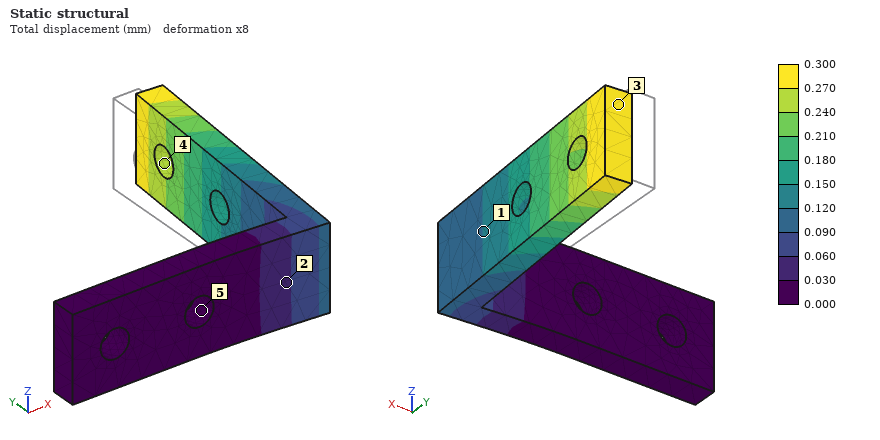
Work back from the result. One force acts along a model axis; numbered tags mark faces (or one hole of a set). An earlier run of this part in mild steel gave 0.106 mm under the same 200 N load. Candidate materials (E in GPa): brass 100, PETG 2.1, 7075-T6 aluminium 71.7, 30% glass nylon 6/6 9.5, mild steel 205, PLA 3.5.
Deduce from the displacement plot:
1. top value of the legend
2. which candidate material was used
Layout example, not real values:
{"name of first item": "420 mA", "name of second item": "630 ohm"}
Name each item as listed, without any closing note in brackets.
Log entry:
{"top value of the legend": "0.300 mm", "which candidate material was used": "7075-T6 aluminium"}
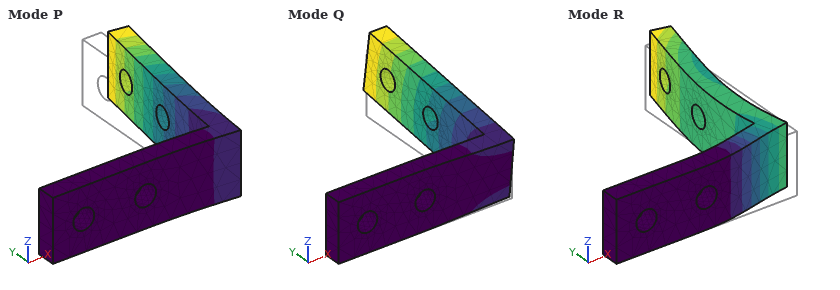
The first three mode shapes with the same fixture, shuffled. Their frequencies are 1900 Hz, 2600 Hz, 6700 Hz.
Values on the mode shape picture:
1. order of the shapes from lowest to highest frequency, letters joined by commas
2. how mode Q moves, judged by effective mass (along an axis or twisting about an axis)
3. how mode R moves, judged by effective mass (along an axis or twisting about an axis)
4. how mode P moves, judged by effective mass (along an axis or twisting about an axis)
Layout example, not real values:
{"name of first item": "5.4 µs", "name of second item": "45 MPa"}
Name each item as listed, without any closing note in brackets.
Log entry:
{"order of the shapes from lowest to highest frequency, letters joined by commas": "P, Q, R", "how mode Q moves, judged by effective mass": "along Z", "how mode R moves, judged by effective mass": "along Y", "how mode P moves, judged by effective mass": "along X"}
